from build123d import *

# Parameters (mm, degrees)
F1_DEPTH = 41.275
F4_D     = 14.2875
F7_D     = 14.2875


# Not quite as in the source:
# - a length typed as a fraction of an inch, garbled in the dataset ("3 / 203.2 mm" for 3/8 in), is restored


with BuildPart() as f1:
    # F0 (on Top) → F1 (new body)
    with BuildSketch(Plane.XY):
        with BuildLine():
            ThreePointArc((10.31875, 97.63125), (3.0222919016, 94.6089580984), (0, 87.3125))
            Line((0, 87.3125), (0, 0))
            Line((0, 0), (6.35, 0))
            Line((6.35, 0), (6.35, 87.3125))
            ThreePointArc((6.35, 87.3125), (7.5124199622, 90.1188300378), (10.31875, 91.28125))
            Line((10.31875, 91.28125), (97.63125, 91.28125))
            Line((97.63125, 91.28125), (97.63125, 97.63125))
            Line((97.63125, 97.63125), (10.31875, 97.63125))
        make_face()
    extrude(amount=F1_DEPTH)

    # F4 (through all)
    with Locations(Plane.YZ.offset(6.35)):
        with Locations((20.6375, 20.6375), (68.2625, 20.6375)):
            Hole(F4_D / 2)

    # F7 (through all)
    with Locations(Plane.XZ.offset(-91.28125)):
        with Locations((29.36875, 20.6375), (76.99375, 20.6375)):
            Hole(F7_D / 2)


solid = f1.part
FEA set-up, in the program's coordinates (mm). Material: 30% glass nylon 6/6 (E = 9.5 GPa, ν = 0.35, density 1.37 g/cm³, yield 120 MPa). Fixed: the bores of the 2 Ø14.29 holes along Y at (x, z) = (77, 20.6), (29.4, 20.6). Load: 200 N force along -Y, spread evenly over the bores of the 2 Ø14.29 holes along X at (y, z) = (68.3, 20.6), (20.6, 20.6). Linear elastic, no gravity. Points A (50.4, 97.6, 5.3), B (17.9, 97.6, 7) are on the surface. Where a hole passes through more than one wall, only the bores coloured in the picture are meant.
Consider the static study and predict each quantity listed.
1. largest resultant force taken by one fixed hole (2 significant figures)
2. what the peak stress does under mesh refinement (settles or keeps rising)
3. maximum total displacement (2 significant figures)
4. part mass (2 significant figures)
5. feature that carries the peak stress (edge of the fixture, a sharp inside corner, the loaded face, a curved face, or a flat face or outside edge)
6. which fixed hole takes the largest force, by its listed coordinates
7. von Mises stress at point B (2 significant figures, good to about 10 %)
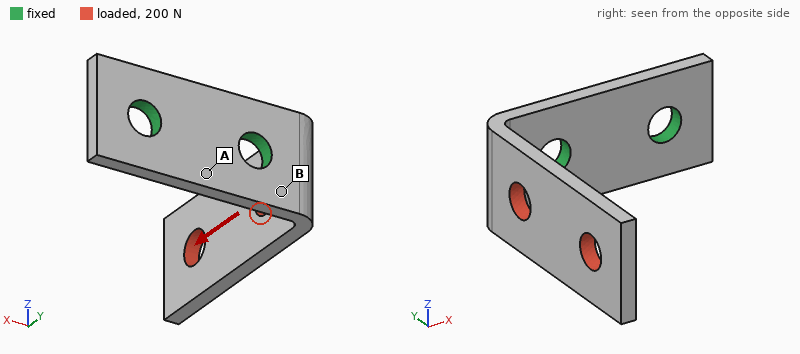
200 N
keeps rising
0.54 mm
61 g
edge of the fixture
(29.4, 20.6)
7.7 MPa
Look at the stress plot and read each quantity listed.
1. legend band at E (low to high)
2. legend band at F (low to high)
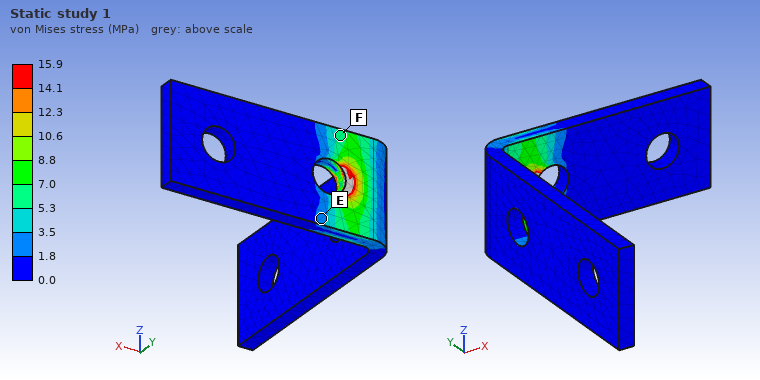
1.8 to 3.5 MPa
5.3 to 7.0 MPa
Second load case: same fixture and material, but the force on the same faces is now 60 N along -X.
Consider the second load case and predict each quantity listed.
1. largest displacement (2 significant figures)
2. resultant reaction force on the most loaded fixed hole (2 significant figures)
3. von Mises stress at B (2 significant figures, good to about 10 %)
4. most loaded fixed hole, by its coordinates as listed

1.5 mm
58 N
8.7 MPa
(29.4, 20.6)
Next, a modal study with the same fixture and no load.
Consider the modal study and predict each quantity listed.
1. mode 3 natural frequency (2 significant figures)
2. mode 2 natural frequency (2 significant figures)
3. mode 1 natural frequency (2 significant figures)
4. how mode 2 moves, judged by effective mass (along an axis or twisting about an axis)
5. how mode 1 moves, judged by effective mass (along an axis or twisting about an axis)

1200 Hz
440 Hz
230 Hz
along Z
along X
